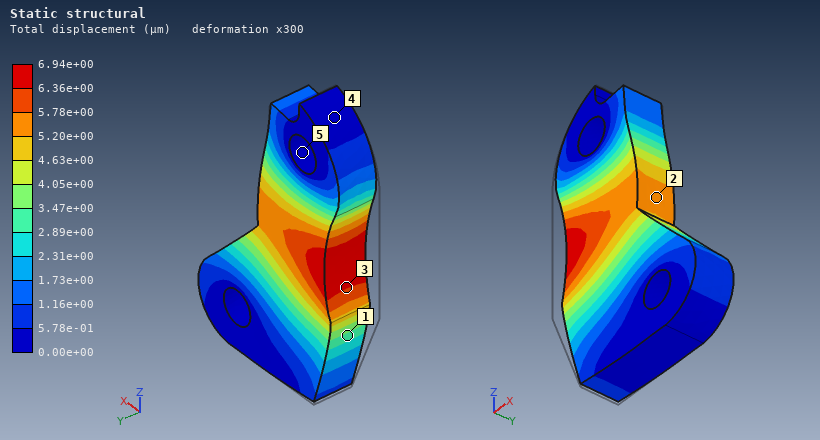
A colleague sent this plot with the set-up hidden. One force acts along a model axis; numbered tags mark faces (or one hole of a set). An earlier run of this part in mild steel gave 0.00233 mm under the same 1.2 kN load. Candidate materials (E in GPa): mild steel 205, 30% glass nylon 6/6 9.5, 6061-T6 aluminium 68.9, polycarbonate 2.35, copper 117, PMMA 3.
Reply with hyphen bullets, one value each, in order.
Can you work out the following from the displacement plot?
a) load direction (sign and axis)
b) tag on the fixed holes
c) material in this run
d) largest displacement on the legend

- +X
- 5
- 6061-T6 aluminium
- 6.94e+00 µm
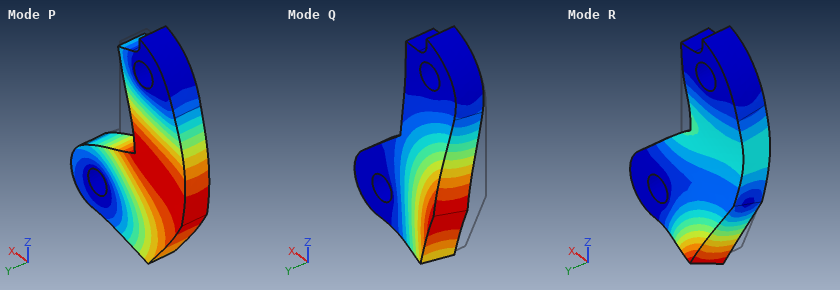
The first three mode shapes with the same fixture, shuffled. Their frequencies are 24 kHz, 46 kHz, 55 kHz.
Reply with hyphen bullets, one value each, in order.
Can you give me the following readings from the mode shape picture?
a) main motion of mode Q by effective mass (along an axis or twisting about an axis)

- along Y
